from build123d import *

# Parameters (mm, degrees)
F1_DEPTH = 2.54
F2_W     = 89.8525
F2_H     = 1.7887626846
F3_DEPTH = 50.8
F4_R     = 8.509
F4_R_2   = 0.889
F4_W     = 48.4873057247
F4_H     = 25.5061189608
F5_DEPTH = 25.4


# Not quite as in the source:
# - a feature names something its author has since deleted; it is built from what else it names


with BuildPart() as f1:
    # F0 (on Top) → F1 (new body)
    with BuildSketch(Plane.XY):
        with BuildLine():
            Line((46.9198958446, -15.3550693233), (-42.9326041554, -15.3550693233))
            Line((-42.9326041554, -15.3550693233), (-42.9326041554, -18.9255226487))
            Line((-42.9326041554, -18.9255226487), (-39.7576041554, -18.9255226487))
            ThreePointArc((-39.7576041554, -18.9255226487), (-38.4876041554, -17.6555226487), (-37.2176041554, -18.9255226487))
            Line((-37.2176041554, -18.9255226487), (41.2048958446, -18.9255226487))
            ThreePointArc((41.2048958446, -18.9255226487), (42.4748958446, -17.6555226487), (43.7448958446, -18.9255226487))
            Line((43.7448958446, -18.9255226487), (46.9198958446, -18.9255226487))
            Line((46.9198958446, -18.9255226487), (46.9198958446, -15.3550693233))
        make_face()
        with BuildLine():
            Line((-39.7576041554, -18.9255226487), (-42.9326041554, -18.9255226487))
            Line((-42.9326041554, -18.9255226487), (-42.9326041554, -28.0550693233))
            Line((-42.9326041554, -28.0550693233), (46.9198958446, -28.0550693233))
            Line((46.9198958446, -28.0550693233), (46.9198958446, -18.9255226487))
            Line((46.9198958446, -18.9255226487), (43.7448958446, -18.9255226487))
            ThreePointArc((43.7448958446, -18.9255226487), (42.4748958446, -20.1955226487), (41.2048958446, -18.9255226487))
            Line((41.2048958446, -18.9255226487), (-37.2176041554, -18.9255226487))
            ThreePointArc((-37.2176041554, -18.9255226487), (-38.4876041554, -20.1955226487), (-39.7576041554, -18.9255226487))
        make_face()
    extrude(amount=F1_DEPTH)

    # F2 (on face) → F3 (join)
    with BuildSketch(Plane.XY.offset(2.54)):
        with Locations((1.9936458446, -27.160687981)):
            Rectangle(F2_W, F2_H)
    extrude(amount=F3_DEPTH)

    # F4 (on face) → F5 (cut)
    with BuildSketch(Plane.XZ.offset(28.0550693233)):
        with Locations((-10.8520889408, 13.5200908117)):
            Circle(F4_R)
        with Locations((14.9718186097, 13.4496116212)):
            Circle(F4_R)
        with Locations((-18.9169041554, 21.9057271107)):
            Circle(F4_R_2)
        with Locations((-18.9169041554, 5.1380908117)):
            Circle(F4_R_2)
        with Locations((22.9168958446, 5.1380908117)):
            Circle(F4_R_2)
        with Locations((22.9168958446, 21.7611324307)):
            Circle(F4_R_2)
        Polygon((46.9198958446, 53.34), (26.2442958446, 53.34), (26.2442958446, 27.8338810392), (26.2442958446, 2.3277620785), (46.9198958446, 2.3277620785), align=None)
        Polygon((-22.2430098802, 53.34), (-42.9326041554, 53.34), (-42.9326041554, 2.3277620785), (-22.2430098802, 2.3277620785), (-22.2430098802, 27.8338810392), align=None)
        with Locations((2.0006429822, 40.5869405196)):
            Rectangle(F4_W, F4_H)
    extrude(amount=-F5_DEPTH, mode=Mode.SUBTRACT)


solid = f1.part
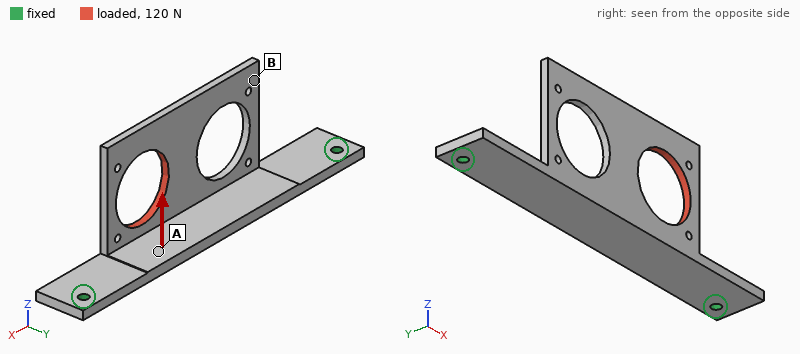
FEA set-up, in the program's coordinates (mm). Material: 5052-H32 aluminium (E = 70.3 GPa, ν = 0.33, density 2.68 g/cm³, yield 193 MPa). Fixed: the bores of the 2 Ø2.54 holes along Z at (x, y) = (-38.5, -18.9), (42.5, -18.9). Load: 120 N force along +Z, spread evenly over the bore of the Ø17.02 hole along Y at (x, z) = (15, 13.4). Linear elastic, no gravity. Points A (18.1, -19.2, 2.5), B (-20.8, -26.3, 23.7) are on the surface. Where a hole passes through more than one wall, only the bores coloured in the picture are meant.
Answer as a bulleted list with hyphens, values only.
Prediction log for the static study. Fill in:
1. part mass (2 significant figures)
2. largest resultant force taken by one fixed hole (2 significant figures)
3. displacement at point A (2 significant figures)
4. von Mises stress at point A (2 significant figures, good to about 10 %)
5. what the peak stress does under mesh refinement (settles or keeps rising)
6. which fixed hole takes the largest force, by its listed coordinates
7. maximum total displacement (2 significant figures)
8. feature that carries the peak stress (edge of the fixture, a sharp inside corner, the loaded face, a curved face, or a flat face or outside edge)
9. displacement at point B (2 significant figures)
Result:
- 11 g
- 87 N
- 0.062 mm
- 17 MPa
- keeps rising
- (42.5, -18.9)
- 0.18 mm
- edge of the fixture
- 0.11 mm
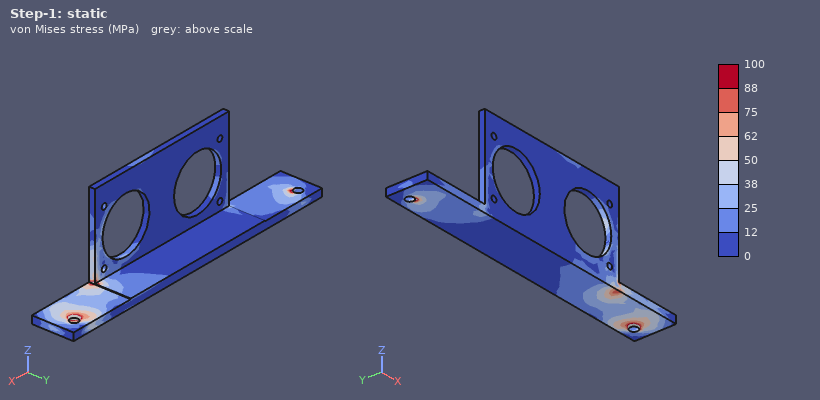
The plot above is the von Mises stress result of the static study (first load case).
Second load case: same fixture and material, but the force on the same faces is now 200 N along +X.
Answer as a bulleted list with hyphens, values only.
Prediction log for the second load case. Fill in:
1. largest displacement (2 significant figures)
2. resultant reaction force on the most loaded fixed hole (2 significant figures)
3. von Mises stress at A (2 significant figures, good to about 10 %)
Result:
- 62 µm
- 110 N
- 11 MPa
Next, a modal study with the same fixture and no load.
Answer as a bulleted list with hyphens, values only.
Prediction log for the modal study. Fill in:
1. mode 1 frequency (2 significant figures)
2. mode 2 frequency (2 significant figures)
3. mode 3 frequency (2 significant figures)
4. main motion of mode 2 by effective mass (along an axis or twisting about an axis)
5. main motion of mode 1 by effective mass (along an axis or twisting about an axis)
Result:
- 1100 Hz
- 2300 Hz
- 2600 Hz
- along Z
- along Y
